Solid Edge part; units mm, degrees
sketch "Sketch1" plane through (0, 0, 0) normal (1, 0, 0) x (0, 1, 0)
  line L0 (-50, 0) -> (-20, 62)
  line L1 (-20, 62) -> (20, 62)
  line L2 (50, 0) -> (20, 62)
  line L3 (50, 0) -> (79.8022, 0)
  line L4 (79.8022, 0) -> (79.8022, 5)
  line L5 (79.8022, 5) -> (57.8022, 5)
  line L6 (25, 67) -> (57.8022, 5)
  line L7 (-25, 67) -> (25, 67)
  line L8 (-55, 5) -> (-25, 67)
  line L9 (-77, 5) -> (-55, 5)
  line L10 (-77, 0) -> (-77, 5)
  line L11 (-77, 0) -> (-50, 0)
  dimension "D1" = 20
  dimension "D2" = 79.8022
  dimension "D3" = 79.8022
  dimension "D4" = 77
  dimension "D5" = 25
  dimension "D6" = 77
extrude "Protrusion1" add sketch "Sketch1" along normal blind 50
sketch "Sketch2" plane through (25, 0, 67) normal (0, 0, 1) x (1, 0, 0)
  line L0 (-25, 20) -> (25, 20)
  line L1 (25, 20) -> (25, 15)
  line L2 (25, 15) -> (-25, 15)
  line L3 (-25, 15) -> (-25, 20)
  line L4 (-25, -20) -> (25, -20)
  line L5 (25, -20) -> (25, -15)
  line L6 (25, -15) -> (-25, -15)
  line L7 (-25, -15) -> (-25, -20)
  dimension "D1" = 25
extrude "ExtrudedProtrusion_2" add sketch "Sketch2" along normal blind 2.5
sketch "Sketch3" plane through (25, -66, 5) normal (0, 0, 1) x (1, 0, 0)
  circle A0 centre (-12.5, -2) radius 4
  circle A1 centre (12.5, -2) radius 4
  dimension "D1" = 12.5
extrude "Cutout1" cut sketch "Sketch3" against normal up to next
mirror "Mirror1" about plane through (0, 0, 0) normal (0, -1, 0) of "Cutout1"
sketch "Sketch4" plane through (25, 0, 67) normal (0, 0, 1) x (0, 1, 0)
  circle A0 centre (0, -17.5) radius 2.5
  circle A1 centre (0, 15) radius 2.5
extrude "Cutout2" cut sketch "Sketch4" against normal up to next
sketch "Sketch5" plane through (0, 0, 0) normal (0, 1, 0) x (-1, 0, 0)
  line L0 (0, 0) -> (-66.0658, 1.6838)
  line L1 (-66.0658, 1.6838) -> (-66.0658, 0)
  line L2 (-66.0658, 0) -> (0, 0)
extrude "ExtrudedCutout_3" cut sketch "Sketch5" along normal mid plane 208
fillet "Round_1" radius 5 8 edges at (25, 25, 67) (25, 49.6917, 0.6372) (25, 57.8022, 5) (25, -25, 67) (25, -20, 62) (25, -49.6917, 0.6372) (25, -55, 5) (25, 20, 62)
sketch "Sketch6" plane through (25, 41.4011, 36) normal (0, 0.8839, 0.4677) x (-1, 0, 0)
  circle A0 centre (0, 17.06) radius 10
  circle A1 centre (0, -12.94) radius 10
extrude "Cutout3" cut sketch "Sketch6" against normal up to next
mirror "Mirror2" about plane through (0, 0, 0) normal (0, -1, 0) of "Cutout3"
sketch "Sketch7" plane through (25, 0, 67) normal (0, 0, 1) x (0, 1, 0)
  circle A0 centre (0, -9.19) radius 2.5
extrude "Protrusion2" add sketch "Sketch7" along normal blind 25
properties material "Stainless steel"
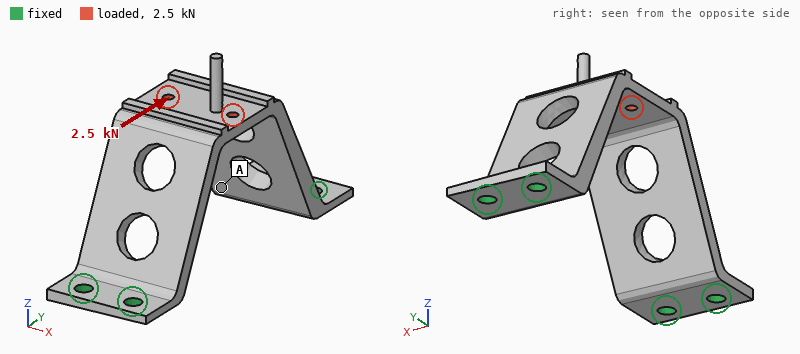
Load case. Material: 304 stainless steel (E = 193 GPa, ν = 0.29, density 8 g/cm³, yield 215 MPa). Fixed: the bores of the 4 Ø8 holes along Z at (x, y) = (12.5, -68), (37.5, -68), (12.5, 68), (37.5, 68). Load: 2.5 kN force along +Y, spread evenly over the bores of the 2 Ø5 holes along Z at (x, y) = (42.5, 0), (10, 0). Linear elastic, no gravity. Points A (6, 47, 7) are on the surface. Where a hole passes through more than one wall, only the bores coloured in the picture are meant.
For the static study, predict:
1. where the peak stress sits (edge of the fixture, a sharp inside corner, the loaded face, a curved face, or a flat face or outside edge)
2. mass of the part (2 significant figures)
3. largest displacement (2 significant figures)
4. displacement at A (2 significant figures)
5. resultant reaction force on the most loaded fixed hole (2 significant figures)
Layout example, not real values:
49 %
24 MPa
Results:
a curved face
510 g
0.10 mm
0.017 mm
890 N
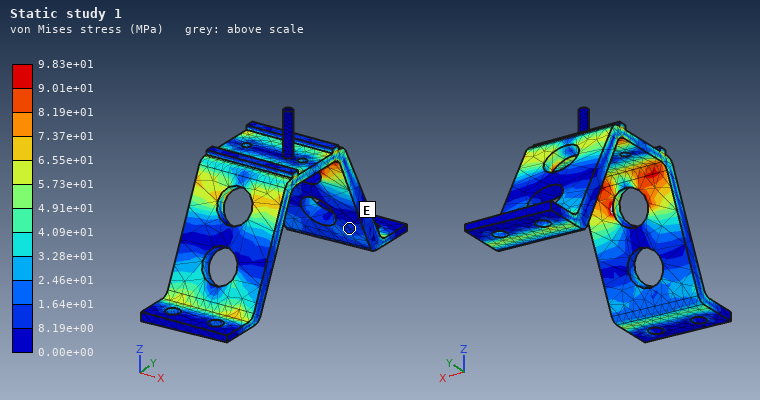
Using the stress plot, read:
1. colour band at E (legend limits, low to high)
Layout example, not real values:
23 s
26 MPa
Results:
8.19e+00 to 1.64e+01 MPa
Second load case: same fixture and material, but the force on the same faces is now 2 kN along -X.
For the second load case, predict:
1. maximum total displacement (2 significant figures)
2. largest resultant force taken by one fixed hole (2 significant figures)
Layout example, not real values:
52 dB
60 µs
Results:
0.12 mm
3.1 kN
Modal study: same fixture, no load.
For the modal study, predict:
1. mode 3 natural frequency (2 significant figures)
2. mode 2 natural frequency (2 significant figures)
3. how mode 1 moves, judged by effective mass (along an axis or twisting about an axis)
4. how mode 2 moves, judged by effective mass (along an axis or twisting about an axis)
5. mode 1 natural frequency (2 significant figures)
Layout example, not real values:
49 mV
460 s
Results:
2500 Hz
1600 Hz
along Y
along X
1500 Hz
